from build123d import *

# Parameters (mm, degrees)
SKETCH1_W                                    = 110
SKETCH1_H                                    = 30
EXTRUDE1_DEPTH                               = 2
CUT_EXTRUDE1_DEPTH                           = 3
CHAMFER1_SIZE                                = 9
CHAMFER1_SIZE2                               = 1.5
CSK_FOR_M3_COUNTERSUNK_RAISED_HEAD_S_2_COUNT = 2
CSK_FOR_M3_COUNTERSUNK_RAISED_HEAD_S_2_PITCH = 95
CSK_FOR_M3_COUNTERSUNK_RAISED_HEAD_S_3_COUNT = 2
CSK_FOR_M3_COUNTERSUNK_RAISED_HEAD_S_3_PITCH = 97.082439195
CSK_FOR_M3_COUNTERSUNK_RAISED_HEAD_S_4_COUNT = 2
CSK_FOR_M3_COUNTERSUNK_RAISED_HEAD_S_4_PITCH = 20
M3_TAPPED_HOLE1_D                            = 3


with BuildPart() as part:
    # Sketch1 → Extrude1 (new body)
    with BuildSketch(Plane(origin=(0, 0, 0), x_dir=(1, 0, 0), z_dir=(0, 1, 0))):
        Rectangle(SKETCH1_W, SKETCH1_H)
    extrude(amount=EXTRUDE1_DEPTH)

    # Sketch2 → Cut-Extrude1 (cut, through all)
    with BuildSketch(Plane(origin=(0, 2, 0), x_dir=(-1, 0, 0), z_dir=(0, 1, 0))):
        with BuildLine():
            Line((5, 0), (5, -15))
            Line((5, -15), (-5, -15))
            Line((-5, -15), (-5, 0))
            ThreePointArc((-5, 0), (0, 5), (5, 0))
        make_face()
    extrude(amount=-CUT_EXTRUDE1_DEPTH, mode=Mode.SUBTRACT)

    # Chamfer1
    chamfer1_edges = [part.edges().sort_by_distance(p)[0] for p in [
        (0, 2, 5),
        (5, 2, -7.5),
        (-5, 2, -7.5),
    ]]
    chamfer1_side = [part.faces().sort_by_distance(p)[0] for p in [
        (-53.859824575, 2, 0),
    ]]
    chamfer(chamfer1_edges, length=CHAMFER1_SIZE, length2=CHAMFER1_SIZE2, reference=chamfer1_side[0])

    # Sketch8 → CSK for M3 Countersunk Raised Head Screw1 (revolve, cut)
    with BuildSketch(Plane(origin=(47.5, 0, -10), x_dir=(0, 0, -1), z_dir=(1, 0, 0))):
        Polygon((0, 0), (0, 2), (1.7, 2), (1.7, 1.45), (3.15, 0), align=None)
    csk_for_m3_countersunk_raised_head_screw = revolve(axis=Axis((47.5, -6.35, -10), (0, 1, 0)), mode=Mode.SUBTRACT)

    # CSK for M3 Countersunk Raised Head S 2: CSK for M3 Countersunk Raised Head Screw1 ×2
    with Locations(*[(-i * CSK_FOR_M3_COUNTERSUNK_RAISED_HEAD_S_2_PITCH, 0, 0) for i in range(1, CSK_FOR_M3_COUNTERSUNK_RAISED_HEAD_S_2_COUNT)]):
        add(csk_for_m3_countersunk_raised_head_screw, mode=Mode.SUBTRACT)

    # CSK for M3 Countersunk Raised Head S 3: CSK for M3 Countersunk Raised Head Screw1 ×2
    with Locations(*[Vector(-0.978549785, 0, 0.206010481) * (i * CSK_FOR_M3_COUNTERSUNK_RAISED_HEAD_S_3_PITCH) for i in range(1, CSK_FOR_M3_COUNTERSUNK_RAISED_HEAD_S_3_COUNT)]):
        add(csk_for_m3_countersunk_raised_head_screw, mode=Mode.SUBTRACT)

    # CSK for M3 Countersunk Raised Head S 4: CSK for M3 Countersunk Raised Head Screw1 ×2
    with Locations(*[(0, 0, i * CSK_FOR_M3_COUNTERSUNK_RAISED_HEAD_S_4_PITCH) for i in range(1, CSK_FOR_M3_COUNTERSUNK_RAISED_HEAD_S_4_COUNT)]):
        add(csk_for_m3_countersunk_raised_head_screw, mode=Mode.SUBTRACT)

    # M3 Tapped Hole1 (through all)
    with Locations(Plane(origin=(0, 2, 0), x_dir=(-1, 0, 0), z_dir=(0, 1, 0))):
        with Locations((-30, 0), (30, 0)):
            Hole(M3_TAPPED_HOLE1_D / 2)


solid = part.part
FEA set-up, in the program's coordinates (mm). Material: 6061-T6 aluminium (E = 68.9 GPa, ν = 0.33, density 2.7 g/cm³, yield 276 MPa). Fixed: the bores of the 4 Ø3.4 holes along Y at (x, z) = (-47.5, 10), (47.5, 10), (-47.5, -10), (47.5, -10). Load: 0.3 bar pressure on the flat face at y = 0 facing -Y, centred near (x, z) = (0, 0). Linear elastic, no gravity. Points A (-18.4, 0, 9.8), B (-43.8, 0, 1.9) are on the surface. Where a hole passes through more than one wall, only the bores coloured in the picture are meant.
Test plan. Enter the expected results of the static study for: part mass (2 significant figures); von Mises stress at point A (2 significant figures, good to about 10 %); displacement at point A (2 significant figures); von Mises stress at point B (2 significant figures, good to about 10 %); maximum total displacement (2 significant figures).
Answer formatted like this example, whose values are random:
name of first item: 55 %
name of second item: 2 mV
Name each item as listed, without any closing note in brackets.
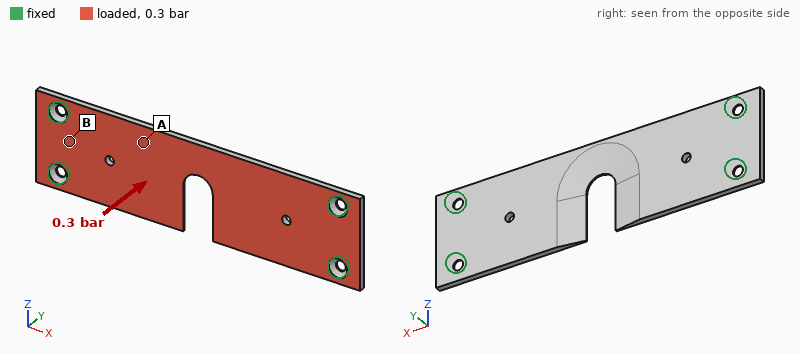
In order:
part mass: 15 g
von Mises stress at point A: 10 MPa
displacement at point A: 0.16 mm
von Mises stress at point B: 23 MPa
maximum total displacement: 0.27 mm
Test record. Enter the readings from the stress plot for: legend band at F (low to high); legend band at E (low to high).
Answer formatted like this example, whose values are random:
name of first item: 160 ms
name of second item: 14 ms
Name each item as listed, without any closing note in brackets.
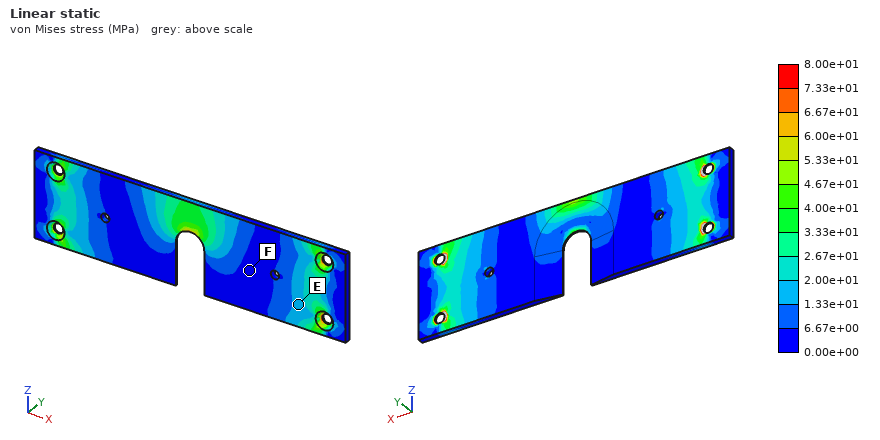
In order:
legend band at F: 0.00e+00 to 6.67e+00 MPa
legend band at E: 1.33e+01 to 2.00e+01 MPa
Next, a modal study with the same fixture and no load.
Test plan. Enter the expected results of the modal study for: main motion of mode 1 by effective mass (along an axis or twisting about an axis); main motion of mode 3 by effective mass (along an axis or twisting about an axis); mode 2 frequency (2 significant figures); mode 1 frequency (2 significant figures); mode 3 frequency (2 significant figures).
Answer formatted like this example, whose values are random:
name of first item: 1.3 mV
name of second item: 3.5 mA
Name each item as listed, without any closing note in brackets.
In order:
main motion of mode 1 by effective mass: along Y
main motion of mode 3 by effective mass: twisting about X
mode 2 frequency: 2000 Hz
mode 1 frequency: 990 Hz
mode 3 frequency: 2700 Hz
